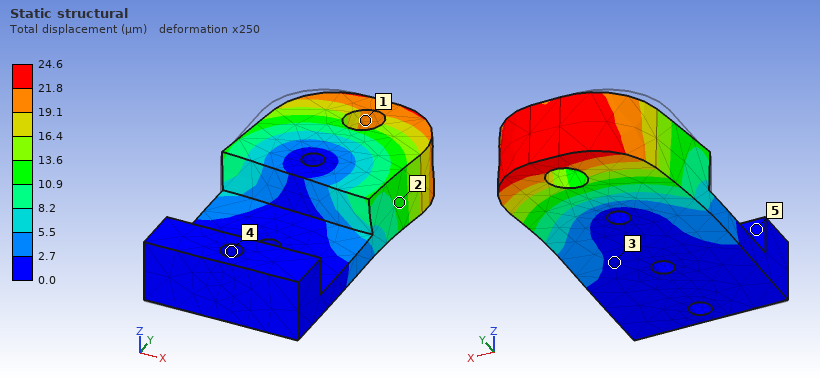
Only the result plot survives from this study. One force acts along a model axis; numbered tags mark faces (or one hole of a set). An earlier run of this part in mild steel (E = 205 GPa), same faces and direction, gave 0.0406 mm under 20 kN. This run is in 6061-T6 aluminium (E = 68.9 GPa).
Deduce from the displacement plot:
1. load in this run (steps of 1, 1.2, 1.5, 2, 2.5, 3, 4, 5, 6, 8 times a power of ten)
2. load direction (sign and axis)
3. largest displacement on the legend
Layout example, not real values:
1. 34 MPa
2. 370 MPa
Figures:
1. 4 kN
2. +X
3. 24.6 µm
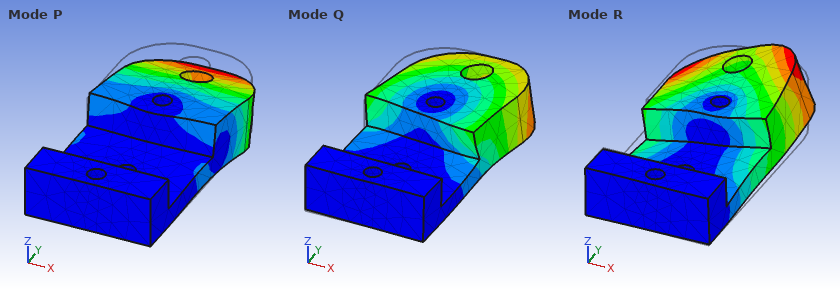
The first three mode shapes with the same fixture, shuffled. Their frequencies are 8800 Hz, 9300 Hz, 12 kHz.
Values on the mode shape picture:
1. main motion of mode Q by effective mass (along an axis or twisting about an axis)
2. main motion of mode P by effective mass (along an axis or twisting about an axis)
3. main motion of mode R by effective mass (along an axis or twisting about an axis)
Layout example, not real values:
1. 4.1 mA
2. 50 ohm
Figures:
1. along X
2. along Z
3. twisting about Y
